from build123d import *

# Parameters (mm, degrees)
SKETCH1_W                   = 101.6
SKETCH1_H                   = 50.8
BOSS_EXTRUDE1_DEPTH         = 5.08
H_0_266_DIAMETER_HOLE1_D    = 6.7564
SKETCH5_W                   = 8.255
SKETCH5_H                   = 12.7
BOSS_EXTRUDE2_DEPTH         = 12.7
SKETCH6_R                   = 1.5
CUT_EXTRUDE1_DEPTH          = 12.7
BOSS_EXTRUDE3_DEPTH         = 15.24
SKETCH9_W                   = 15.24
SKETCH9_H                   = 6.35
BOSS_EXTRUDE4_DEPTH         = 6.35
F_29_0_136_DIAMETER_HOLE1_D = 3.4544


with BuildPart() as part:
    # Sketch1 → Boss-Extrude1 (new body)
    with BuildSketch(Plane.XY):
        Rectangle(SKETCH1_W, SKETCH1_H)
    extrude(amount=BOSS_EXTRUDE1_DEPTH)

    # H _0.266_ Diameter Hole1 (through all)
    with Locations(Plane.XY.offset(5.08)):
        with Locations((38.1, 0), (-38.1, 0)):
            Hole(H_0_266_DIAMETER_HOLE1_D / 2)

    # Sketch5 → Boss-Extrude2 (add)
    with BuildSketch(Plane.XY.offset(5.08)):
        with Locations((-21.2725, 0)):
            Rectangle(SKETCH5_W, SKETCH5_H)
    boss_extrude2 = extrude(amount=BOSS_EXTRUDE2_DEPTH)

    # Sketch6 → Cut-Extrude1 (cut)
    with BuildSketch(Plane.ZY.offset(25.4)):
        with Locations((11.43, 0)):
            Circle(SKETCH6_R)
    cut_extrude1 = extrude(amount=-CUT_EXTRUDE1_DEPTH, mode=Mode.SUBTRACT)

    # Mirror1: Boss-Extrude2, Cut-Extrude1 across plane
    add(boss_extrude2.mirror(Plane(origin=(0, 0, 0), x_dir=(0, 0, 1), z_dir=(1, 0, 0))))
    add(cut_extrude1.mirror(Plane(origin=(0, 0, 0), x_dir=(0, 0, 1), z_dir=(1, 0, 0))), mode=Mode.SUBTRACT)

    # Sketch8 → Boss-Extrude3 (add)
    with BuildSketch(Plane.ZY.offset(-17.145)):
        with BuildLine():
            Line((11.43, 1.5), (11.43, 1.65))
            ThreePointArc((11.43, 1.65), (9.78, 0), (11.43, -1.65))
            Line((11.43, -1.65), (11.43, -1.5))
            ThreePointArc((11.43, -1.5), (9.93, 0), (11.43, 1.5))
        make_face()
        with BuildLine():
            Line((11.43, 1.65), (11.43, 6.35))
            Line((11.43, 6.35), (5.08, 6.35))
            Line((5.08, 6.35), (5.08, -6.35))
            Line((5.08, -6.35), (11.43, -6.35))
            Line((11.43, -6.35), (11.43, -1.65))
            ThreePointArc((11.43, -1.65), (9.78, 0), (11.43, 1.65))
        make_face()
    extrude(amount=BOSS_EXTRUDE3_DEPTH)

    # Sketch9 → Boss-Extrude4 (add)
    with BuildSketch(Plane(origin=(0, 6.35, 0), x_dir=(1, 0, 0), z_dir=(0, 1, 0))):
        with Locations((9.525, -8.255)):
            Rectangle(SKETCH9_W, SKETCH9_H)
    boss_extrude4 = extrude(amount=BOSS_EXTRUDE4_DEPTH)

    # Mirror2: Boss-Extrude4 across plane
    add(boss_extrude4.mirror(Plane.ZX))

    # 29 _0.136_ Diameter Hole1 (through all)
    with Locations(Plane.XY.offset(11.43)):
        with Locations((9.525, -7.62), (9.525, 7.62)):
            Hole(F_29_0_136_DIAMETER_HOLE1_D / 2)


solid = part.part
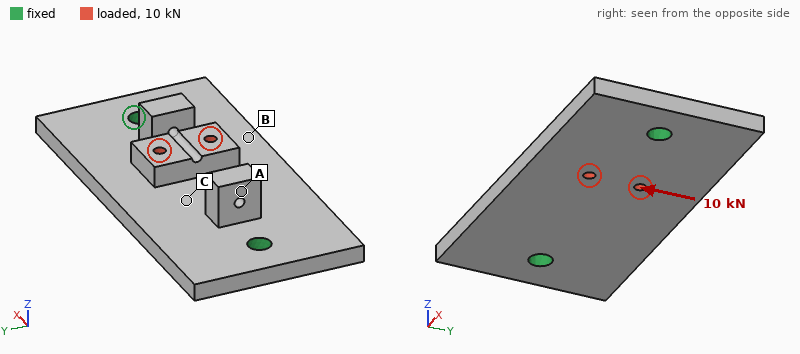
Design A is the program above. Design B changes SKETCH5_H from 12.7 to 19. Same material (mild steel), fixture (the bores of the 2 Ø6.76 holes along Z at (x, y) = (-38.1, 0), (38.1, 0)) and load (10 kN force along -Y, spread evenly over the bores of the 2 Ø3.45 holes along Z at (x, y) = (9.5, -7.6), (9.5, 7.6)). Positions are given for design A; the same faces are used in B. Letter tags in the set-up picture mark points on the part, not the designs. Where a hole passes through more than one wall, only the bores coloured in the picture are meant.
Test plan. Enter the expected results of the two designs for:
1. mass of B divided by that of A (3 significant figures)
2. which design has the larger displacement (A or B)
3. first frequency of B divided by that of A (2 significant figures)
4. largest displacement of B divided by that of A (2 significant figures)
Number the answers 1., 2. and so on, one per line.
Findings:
1. 1.04
2. A
3. 0.99
4. 0.91
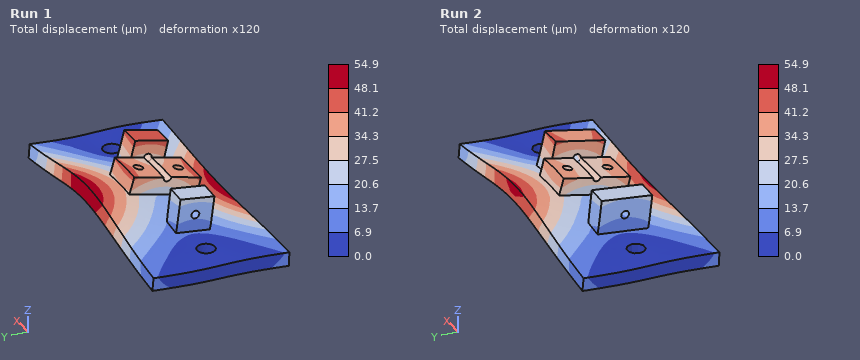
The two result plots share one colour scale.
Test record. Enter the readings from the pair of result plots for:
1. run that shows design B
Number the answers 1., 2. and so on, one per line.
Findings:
1. Run 2
